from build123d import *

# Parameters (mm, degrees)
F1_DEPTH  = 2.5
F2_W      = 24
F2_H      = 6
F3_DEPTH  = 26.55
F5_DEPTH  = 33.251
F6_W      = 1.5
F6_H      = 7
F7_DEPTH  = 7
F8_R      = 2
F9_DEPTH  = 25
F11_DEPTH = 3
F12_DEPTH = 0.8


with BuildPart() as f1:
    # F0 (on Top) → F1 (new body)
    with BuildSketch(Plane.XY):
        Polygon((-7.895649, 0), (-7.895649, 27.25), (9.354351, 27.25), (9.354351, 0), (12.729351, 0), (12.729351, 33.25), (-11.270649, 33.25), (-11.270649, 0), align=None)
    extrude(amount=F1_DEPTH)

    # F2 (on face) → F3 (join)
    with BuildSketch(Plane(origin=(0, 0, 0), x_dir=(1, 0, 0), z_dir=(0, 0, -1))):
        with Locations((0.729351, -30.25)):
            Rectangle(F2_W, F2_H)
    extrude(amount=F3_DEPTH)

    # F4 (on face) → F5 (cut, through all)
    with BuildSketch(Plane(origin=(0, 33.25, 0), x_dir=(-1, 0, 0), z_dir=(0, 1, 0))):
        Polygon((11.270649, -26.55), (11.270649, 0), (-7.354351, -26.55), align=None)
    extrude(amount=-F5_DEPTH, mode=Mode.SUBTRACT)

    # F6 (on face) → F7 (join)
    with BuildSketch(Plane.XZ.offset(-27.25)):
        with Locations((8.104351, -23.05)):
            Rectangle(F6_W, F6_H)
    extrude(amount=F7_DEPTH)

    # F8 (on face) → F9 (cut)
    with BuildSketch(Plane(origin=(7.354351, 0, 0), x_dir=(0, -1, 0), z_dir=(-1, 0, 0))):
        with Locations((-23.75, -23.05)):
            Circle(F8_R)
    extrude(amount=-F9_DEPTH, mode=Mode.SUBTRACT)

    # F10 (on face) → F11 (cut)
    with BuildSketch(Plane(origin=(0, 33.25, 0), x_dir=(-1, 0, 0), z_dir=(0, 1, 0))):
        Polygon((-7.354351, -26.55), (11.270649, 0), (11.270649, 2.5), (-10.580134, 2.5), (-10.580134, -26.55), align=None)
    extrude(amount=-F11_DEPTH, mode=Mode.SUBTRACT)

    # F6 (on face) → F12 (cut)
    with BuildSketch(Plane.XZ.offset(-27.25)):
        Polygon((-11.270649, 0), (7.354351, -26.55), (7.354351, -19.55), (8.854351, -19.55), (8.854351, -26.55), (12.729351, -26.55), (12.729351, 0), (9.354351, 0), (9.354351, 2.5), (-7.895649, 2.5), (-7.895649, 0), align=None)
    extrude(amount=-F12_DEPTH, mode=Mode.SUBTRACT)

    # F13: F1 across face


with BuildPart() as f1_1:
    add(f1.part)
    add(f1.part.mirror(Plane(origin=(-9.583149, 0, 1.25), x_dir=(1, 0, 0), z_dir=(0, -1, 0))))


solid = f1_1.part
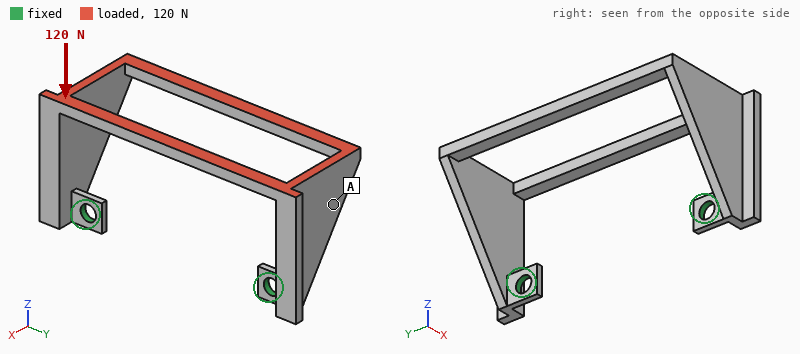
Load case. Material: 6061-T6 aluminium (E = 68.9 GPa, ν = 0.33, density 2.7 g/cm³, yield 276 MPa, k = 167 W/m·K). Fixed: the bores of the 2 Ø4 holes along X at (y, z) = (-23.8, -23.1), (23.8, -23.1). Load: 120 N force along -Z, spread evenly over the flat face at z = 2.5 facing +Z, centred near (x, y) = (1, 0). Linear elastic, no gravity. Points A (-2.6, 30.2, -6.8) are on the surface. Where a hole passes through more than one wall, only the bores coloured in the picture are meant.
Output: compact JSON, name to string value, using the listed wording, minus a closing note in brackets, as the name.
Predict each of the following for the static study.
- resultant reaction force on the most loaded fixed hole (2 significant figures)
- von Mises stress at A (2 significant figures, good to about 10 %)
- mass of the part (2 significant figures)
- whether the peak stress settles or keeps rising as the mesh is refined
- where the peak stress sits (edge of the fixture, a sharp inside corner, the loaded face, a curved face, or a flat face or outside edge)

{"resultant reaction force on the most loaded fixed hole": "62 N", "von Mises stress at A": "14 MPa", "mass of the part": "9.3 g", "whether the peak stress settles or keeps rising as the mesh is refined": "keeps rising", "where the peak stress sits": "edge of the fixture"}
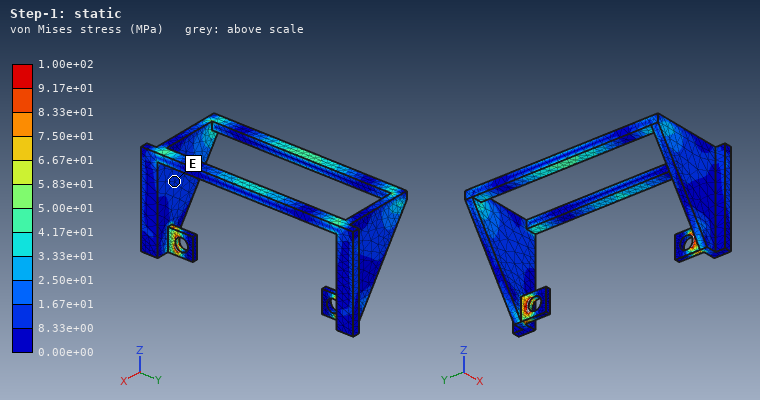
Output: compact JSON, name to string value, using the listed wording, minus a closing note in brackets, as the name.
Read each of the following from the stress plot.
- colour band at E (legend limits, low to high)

{"colour band at E": "8.33e+00 to 1.67e+01 MPa"}
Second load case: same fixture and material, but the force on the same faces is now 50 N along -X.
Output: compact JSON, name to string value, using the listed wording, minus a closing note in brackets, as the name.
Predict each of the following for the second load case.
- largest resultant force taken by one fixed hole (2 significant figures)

{"largest resultant force taken by one fixed hole": "25 N"}
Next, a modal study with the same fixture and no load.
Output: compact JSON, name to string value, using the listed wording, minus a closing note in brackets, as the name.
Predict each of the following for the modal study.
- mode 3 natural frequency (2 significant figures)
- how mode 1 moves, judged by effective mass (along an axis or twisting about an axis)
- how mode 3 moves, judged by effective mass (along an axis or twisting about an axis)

{"mode 3 natural frequency": "1900 Hz", "how mode 1 moves, judged by effective mass": "along X", "how mode 3 moves, judged by effective mass": "along Y"}
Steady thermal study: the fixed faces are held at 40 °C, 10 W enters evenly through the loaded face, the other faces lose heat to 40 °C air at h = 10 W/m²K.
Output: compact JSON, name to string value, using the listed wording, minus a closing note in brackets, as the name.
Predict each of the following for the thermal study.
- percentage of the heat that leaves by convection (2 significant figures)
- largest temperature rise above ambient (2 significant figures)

{"percentage of the heat that leaves by convection": "8.9 %", "largest temperature rise above ambient": "51 K"}
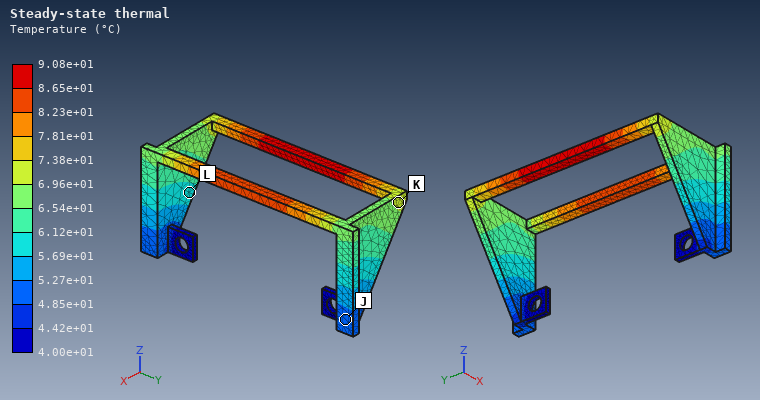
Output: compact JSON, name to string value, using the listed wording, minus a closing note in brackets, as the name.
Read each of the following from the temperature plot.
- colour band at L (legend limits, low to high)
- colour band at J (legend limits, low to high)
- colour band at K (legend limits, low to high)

{"colour band at L": "5.69e+01 to 6.12e+01 °C", "colour band at J": "4.85e+01 to 5.27e+01 °C", "colour band at K": "6.96e+01 to 7.38e+01 °C"}
